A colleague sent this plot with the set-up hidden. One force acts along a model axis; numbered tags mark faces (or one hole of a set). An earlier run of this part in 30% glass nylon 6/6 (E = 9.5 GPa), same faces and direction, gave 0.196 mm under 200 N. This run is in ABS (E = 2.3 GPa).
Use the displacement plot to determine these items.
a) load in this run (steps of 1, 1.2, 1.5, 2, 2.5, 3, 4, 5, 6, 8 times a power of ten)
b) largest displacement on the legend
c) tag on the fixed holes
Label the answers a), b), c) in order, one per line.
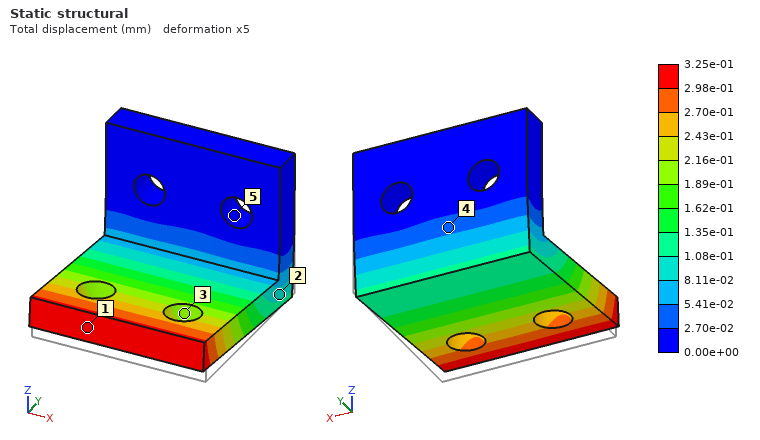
a) 80 N
b) 3.25e-01 mm
c) 5
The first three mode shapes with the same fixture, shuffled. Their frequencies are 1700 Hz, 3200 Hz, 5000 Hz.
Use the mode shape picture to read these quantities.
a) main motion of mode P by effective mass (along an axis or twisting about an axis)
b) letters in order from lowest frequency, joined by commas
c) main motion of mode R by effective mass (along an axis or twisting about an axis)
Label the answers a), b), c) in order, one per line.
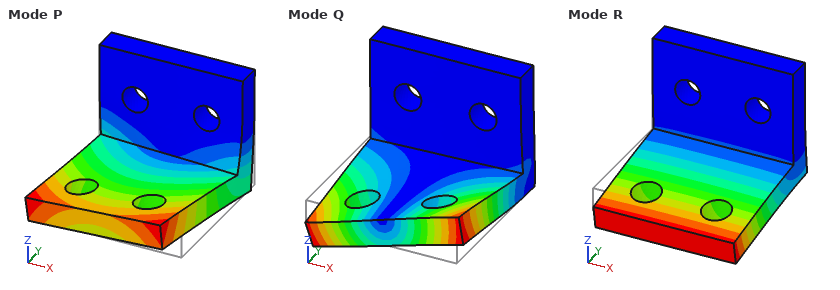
a) along X
b) R, P, Q
c) along Z
